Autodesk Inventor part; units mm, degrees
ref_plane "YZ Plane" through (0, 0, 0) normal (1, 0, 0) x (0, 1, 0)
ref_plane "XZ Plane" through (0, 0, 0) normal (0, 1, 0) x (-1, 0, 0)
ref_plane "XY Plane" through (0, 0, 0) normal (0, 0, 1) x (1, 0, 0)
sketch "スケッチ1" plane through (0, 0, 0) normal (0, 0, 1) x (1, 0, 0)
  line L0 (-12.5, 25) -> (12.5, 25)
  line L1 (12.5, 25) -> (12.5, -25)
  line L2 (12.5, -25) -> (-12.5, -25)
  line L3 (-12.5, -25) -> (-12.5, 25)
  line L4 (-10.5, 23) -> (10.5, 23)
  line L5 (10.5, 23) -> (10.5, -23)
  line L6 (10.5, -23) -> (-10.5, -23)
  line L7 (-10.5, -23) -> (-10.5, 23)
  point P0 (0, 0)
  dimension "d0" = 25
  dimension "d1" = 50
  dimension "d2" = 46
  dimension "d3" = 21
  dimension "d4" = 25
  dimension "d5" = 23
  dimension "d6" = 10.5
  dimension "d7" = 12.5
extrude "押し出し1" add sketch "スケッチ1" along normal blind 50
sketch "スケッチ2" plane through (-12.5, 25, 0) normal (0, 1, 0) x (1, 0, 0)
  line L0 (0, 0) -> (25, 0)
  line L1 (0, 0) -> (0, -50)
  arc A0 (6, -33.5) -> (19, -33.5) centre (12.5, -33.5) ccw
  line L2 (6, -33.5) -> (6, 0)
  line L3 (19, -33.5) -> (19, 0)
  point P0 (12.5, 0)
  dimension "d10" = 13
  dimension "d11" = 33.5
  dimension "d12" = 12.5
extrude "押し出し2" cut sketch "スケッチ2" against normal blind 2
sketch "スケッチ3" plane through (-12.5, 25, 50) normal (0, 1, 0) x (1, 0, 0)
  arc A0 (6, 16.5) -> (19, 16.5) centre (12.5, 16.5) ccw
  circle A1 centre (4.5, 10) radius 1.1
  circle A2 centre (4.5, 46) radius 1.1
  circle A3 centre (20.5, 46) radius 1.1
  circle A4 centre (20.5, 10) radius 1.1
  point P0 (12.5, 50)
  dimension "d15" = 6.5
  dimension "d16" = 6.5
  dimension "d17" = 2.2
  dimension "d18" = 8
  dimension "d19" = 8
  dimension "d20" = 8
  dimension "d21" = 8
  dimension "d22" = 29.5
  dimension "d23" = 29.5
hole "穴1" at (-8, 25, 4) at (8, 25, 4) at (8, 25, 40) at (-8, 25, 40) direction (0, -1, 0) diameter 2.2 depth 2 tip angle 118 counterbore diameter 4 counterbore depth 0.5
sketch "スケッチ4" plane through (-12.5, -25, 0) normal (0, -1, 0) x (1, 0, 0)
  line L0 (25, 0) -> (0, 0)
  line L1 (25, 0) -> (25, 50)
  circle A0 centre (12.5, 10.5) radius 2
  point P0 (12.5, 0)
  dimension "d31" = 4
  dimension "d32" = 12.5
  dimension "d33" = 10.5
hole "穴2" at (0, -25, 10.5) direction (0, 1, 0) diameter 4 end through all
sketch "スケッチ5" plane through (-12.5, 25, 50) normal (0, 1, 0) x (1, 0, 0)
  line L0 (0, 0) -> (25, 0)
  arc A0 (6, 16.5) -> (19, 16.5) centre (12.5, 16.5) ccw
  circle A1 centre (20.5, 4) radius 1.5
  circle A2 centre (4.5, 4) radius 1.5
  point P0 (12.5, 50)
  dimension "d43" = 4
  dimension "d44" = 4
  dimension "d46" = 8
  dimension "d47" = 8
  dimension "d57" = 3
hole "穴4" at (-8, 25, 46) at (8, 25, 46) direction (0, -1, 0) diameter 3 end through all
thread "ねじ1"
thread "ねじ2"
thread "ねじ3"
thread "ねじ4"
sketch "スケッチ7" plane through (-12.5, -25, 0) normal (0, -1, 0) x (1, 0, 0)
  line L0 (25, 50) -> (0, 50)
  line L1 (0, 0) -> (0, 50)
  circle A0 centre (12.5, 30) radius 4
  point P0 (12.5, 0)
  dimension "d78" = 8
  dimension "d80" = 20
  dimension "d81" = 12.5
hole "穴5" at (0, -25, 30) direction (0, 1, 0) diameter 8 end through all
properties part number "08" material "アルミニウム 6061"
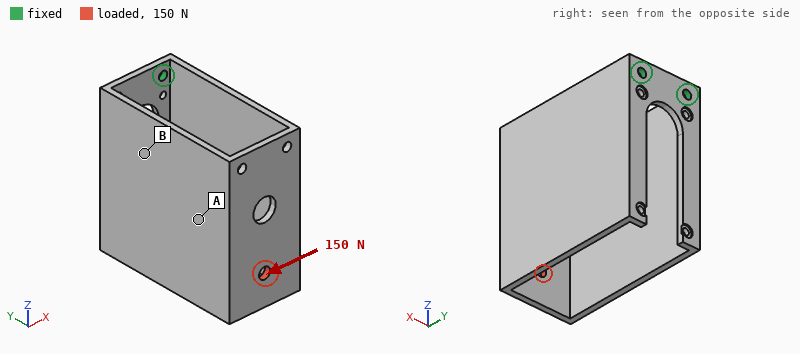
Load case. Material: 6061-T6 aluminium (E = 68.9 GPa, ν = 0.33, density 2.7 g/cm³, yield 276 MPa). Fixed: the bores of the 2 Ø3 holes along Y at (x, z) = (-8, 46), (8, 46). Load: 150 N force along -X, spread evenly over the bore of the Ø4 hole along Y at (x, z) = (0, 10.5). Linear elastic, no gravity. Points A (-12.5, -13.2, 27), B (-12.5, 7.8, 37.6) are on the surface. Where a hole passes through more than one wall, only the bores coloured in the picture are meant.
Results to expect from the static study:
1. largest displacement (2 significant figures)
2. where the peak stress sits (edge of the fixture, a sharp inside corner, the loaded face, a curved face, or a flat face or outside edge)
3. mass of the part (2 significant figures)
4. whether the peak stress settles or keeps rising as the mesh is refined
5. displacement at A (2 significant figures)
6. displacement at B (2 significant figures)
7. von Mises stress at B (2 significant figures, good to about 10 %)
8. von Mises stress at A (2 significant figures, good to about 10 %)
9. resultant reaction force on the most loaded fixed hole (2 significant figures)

0.79 mm
edge of the fixture
35 g
keeps rising
0.62 mm
0.24 mm
15 MPa
38 MPa
360 N
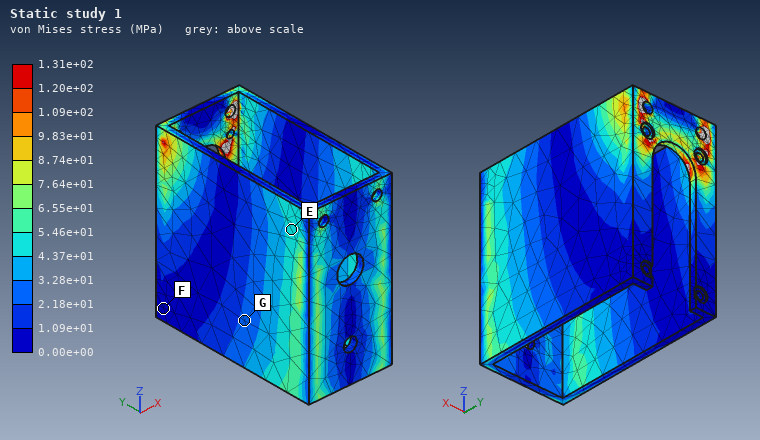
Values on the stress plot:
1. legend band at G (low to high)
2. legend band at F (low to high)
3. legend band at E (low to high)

2.18e+01 to 3.28e+01 MPa
0.00e+00 to 1.09e+01 MPa
4.37e+01 to 5.46e+01 MPa
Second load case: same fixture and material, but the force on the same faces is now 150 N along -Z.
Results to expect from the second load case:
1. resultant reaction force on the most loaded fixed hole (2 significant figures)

76 N
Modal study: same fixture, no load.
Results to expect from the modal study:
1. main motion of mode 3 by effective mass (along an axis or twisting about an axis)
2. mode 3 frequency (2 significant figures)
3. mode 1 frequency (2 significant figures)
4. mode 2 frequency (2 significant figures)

twisting about Y
1100 Hz
560 Hz
570 Hz
